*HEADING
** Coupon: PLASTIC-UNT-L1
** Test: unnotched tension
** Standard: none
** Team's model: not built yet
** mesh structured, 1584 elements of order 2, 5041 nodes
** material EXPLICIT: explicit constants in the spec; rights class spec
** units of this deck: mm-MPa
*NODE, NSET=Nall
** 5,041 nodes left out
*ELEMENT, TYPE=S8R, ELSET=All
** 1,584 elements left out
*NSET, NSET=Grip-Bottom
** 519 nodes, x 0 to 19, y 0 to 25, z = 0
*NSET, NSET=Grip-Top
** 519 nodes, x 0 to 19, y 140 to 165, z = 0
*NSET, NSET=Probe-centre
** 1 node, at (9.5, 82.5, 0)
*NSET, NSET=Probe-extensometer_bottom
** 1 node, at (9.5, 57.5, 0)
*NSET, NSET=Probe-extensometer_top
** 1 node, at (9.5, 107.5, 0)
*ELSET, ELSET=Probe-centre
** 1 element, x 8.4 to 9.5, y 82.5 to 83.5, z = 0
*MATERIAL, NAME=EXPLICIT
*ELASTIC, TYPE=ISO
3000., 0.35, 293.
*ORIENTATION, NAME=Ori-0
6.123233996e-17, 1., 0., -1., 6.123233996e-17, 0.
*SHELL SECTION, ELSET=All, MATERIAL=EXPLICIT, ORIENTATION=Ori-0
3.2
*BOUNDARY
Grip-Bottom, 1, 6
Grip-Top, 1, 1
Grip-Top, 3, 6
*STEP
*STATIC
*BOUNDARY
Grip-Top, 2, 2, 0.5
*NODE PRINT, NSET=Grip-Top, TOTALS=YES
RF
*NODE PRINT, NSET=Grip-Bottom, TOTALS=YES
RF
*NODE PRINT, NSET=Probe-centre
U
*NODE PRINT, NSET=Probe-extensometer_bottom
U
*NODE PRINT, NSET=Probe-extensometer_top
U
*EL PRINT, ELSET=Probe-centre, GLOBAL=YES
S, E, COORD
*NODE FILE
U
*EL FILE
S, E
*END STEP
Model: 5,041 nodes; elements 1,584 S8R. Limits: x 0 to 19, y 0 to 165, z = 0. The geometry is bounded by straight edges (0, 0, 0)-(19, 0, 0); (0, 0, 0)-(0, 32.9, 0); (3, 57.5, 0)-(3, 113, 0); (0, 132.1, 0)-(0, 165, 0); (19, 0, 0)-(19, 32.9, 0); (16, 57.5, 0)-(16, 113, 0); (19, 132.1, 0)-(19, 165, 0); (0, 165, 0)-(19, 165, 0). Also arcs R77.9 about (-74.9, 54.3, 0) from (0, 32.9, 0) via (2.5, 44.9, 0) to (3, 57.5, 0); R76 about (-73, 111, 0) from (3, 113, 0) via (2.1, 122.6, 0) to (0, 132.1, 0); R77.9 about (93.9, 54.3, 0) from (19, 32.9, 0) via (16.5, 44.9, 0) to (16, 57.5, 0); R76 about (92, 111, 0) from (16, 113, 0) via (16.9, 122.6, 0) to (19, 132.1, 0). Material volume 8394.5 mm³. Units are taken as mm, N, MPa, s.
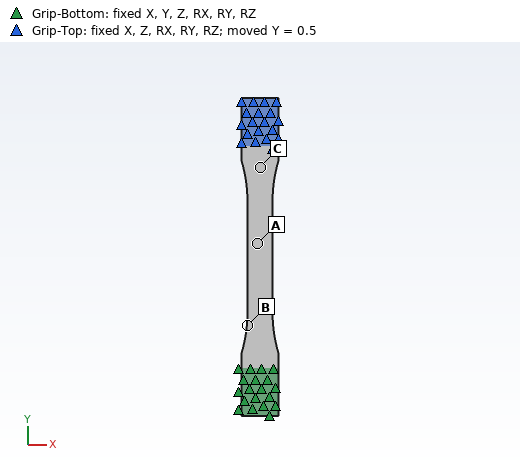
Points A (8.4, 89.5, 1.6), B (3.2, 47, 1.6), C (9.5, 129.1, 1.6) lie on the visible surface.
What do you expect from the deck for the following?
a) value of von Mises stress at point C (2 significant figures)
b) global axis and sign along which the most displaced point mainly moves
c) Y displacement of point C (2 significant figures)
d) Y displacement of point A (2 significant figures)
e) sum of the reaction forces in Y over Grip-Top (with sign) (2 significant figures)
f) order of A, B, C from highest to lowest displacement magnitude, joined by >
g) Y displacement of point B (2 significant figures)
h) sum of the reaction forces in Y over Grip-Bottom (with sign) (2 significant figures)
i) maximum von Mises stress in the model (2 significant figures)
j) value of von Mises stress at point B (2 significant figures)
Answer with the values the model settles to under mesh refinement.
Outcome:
12 MPa
+Y
0.46 mm
0.28 mm
600 N
C > A > B
0.080 mm
-600 N
15 MPa
14 MPa
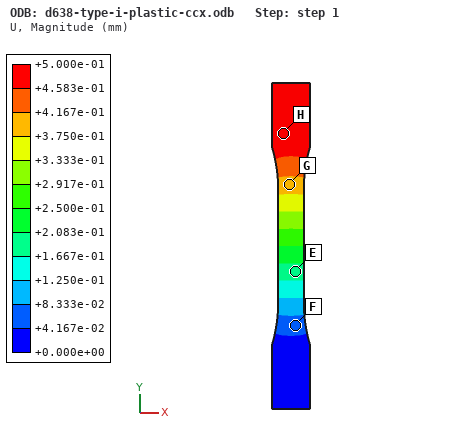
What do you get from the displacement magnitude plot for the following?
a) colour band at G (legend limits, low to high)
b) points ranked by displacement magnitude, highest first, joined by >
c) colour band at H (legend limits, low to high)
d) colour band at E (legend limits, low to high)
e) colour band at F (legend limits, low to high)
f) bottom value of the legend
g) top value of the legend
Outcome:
+3.750e-01 to +4.167e-01 mm
H > G > E > F
+4.583e-01 to +5.000e-01 mm
+1.667e-01 to +2.083e-01 mm
+4.167e-02 to +8.333e-02 mm
+0.000e+00 mm
+5.000e-01 mm
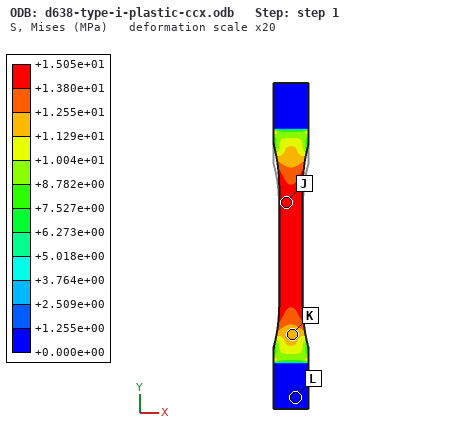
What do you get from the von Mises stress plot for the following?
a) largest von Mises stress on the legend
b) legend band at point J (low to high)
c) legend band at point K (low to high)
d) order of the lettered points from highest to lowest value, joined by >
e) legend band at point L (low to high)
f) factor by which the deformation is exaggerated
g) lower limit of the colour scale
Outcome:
+1.505e+01 MPa
+1.380e+01 to +1.505e+01 MPa
+1.129e+01 to +1.255e+01 MPa
J > K > L
+0.000e+00 to +1.255e+00 MPa
20
+0.000e+00 MPa
